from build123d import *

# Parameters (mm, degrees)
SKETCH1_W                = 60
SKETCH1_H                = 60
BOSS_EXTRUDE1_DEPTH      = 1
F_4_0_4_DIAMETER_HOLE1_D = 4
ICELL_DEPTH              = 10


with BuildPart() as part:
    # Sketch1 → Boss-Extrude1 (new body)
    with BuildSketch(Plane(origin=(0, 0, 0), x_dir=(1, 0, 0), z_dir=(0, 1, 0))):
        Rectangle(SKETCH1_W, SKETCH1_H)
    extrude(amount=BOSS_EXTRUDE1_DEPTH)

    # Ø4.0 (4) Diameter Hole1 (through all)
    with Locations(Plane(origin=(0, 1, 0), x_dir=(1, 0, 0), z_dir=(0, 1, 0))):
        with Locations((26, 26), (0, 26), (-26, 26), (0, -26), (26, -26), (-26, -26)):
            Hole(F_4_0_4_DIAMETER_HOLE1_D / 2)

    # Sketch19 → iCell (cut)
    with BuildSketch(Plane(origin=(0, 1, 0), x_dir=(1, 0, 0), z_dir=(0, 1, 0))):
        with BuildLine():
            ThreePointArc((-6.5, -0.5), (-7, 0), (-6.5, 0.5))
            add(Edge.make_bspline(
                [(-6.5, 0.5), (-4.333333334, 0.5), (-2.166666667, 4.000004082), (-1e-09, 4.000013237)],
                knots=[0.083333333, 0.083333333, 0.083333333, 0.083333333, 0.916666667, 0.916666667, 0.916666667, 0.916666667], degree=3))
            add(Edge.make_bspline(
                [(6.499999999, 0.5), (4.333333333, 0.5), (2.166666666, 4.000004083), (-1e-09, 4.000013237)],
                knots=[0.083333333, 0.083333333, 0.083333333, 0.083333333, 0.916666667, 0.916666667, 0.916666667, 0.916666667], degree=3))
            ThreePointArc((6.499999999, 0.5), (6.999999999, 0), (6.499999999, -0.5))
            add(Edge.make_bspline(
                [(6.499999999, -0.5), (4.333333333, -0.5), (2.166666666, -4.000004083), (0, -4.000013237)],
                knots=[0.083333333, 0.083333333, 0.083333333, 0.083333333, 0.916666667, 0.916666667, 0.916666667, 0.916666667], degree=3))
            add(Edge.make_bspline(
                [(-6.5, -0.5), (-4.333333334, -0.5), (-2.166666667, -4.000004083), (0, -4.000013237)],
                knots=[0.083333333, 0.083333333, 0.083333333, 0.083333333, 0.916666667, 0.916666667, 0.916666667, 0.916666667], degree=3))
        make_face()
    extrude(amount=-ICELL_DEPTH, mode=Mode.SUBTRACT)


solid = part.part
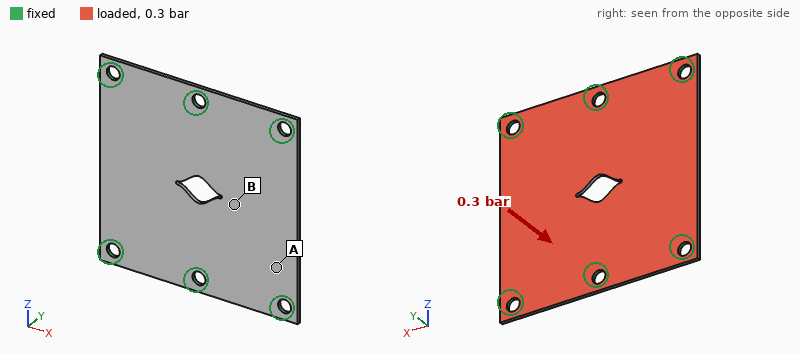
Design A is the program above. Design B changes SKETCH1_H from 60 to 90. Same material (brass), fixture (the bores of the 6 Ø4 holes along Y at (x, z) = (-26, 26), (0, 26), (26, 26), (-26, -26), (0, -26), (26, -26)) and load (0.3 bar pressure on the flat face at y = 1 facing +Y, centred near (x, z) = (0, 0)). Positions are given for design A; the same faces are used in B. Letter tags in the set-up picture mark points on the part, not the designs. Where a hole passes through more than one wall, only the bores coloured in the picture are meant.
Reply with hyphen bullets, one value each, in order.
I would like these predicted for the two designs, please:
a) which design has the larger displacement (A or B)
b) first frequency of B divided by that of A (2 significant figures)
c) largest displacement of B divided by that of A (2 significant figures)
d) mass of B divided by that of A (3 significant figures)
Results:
- A
- 1.00
- 0.89
- 1.52
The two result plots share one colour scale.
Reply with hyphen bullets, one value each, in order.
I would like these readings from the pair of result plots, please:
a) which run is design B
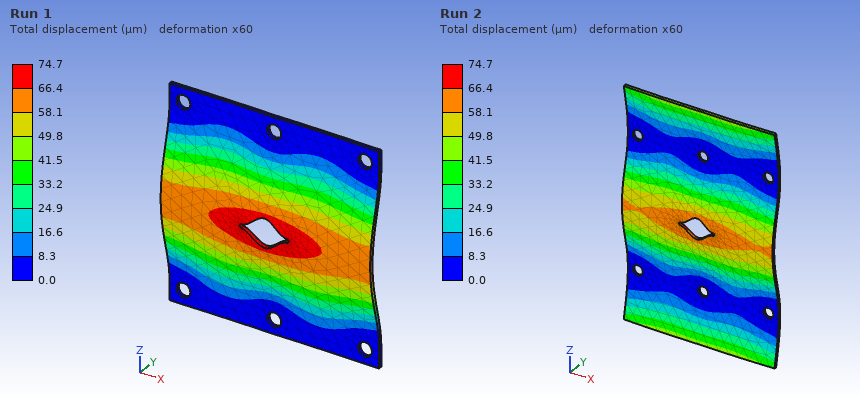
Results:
- Run 2
